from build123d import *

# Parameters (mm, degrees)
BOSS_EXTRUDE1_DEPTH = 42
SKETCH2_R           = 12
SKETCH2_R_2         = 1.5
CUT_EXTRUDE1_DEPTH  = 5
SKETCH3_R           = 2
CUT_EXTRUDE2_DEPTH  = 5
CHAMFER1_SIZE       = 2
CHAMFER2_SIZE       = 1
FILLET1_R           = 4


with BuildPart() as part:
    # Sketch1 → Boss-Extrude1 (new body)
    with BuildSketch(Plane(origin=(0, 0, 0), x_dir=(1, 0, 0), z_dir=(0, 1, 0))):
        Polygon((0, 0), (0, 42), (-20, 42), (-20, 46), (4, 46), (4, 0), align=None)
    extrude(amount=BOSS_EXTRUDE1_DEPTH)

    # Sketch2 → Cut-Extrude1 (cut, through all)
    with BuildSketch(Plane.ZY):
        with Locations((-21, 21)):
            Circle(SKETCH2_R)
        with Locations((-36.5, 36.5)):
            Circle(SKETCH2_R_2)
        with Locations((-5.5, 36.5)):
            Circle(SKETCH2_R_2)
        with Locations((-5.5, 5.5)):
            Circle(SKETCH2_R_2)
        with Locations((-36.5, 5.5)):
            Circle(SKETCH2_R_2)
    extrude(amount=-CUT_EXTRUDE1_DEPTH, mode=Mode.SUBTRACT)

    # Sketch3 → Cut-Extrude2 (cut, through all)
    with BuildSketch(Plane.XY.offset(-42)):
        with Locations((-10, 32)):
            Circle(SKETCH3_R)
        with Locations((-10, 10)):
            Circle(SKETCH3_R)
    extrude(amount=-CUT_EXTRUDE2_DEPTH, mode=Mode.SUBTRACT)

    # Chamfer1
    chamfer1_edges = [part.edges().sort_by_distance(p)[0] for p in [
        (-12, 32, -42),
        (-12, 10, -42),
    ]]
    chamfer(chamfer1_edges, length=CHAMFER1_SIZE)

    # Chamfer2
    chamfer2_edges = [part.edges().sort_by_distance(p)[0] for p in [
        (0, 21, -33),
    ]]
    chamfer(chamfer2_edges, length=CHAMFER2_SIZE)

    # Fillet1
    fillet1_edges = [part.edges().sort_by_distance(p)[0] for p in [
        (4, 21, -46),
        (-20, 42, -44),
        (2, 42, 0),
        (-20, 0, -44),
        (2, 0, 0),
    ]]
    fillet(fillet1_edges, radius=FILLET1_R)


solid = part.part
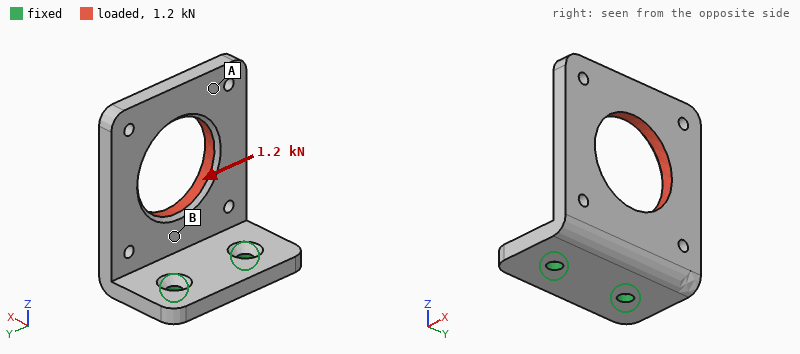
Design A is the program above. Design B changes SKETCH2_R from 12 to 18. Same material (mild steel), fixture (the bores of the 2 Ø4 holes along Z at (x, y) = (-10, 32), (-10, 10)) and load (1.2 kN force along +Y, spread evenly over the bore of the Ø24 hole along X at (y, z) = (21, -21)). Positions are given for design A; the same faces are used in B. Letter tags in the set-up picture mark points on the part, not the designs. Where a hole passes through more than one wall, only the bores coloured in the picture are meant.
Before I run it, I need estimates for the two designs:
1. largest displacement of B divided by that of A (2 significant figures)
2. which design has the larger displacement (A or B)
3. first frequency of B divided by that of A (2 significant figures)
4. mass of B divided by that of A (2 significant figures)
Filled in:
2.0
B
0.97
0.74
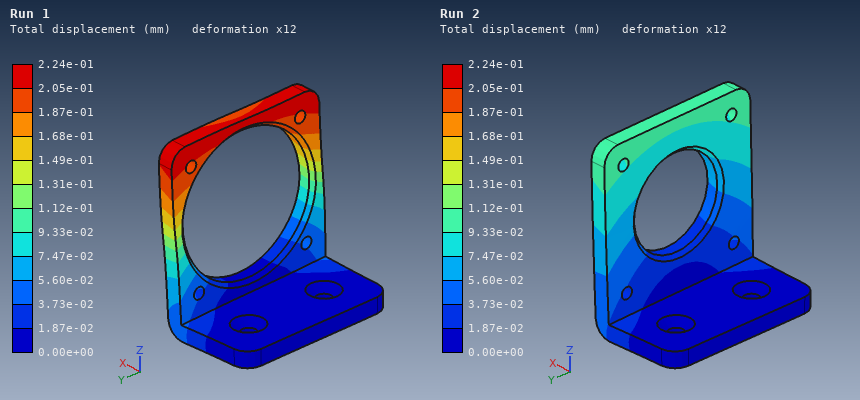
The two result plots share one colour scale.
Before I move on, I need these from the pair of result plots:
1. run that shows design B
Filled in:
Run 1
